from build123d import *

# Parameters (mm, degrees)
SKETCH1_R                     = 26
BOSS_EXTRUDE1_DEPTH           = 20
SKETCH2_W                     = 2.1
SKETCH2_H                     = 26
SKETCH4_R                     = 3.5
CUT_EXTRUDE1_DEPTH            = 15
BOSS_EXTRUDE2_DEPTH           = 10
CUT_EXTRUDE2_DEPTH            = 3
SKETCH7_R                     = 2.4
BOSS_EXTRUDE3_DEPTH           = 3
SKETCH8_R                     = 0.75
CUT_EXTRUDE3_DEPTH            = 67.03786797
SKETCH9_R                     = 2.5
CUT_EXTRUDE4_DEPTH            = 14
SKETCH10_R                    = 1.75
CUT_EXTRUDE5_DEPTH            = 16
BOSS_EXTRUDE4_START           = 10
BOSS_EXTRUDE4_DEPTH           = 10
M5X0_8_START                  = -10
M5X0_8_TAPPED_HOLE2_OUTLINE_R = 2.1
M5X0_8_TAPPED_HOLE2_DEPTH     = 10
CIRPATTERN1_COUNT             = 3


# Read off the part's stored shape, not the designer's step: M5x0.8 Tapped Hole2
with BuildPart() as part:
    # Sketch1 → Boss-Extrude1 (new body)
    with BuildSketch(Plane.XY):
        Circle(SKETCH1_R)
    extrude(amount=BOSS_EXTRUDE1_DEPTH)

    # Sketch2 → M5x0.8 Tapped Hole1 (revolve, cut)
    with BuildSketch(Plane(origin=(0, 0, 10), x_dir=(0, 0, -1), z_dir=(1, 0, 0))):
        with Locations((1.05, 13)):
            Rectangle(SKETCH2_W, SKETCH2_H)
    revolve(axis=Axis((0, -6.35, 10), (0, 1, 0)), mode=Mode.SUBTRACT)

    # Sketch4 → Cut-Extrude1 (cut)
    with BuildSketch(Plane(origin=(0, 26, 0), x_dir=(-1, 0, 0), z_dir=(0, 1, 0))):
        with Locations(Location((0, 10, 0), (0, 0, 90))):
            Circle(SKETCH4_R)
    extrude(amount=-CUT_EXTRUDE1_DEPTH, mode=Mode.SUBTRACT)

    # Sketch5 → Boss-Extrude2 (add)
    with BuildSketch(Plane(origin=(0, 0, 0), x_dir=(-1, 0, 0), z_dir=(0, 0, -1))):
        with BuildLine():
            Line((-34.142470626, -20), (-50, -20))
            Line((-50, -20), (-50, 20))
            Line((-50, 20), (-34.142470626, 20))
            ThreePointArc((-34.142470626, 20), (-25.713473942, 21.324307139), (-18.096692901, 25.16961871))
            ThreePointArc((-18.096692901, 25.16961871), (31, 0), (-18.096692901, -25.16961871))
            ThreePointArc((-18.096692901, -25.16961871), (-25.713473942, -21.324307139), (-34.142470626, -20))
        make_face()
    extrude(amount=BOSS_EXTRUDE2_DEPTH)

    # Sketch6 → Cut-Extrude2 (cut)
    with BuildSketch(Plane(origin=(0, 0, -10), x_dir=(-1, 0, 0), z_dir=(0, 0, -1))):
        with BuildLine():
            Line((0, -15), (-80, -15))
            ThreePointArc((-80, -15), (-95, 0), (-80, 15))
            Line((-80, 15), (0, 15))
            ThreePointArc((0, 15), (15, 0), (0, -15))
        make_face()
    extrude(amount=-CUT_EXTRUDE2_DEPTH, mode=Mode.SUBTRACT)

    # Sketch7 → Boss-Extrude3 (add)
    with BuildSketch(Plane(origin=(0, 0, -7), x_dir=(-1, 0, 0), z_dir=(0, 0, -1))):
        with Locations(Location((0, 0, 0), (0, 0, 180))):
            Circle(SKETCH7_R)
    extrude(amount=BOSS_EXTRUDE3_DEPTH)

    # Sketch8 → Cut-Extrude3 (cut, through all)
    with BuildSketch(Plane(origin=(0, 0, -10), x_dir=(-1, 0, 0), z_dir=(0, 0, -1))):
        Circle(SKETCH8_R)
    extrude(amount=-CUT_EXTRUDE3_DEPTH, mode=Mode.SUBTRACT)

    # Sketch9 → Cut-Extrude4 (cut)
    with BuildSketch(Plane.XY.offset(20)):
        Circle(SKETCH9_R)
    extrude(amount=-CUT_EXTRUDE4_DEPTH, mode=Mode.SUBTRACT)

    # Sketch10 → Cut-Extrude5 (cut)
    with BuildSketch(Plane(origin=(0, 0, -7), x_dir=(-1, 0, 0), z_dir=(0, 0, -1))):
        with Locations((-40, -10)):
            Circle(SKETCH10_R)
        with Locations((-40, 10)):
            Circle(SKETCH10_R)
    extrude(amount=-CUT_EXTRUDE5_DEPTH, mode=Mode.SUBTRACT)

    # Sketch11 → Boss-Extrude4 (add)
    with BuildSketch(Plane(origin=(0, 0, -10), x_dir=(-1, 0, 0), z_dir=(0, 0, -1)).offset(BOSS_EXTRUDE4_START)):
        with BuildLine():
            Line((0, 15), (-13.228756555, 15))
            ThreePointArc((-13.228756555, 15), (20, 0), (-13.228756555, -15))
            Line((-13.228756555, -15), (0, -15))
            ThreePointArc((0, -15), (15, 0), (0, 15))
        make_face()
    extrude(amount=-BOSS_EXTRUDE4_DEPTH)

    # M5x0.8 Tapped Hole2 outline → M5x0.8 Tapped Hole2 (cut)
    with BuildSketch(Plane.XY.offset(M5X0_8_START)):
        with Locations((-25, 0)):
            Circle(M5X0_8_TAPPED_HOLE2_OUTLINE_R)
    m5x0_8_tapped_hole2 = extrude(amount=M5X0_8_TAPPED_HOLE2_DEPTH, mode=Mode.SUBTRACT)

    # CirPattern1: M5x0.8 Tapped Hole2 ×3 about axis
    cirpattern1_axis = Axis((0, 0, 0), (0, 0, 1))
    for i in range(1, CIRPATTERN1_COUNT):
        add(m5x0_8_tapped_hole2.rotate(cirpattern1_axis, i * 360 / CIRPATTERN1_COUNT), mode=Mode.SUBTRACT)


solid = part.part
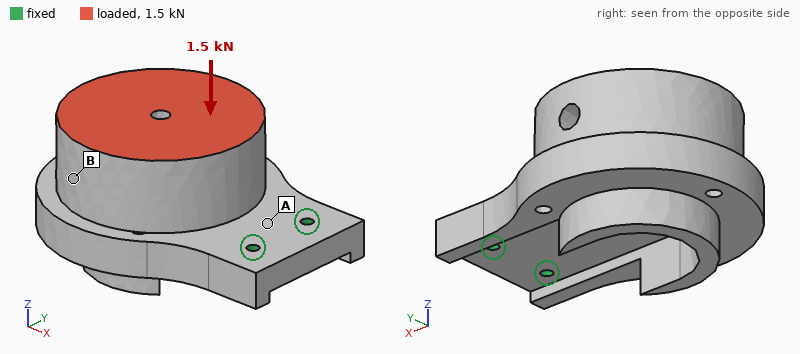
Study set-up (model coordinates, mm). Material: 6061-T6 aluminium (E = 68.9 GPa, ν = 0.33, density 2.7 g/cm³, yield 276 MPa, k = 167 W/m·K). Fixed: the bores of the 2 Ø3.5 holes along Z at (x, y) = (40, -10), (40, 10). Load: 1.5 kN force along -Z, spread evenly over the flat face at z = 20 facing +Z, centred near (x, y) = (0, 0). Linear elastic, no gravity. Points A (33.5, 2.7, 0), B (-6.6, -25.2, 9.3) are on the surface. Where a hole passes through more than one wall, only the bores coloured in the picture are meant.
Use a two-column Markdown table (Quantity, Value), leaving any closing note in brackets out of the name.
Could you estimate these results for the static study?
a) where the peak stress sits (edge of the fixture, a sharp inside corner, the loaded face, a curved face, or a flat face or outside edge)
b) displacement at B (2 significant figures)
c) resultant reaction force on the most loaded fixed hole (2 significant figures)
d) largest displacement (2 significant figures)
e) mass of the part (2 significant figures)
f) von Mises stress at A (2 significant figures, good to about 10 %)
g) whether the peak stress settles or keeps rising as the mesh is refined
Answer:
| Quantity | Value |
|---|---|
| where the peak stress sits | edge of the fixture |
| displacement at B | 0.37 mm |
| resultant reaction force on the most loaded fixed hole | 760 N |
| largest displacement | 0.57 mm |
| mass of the part | 210 g |
| von Mises stress at A | 97 MPa |
| whether the peak stress settles or keeps rising as the mesh is refined | keeps rising |
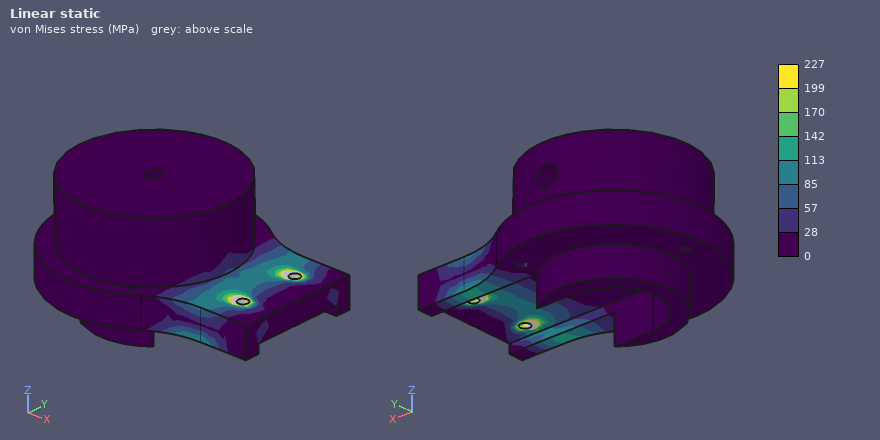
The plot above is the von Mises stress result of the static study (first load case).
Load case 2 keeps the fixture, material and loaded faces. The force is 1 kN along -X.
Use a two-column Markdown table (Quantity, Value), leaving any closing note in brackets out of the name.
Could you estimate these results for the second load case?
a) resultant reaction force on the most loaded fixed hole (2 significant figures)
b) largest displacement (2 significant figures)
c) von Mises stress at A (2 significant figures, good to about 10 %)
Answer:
| Quantity | Value |
|---|---|
| resultant reaction force on the most loaded fixed hole | 520 N |
| largest displacement | 0.28 mm |
| von Mises stress at A | 49 MPa |
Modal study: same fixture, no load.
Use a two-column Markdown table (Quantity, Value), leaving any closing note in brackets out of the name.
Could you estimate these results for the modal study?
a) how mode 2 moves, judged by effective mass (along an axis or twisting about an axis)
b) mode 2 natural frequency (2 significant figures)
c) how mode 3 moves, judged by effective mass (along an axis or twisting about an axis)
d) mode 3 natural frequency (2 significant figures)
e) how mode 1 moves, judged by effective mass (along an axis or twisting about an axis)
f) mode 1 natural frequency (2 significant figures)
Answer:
| Quantity | Value |
|---|---|
| how mode 2 moves, judged by effective mass | along Y |
| mode 2 natural frequency | 2200 Hz |
| how mode 3 moves, judged by effective mass | along Y |
| mode 3 natural frequency | 2800 Hz |
| how mode 1 moves, judged by effective mass | along Z |
| mode 1 natural frequency | 700 Hz |
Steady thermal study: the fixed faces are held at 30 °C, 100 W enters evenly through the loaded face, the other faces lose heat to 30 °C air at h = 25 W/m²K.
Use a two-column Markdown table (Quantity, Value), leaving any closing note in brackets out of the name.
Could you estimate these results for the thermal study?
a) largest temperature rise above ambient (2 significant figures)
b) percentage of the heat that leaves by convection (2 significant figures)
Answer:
| Quantity | Value |
|---|---|
| largest temperature rise above ambient | 50 K |
| percentage of the heat that leaves by convection | 13 % |
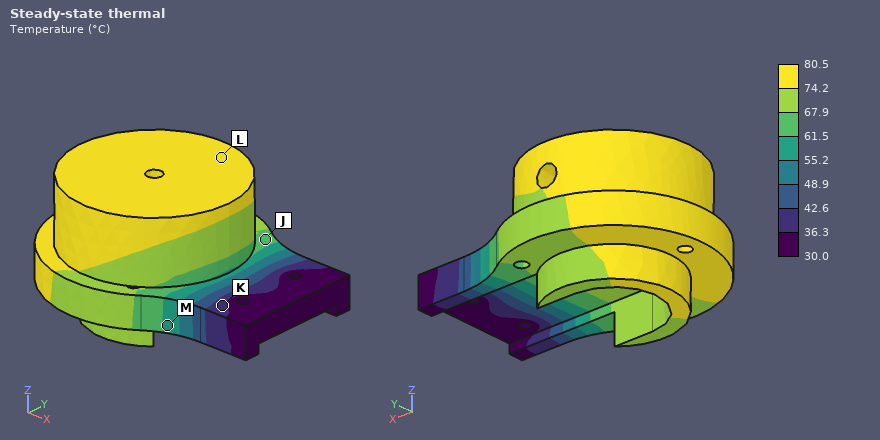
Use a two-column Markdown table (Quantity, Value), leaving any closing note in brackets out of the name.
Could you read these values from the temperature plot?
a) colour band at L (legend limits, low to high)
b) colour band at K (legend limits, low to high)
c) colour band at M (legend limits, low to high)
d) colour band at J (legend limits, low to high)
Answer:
| Quantity | Value |
|---|---|
| colour band at L | 74.2 to 80.5 °C |
| colour band at K | 36.3 to 42.6 °C |
| colour band at M | 55.2 to 61.5 °C |
| colour band at J | 61.5 to 67.9 °C |
